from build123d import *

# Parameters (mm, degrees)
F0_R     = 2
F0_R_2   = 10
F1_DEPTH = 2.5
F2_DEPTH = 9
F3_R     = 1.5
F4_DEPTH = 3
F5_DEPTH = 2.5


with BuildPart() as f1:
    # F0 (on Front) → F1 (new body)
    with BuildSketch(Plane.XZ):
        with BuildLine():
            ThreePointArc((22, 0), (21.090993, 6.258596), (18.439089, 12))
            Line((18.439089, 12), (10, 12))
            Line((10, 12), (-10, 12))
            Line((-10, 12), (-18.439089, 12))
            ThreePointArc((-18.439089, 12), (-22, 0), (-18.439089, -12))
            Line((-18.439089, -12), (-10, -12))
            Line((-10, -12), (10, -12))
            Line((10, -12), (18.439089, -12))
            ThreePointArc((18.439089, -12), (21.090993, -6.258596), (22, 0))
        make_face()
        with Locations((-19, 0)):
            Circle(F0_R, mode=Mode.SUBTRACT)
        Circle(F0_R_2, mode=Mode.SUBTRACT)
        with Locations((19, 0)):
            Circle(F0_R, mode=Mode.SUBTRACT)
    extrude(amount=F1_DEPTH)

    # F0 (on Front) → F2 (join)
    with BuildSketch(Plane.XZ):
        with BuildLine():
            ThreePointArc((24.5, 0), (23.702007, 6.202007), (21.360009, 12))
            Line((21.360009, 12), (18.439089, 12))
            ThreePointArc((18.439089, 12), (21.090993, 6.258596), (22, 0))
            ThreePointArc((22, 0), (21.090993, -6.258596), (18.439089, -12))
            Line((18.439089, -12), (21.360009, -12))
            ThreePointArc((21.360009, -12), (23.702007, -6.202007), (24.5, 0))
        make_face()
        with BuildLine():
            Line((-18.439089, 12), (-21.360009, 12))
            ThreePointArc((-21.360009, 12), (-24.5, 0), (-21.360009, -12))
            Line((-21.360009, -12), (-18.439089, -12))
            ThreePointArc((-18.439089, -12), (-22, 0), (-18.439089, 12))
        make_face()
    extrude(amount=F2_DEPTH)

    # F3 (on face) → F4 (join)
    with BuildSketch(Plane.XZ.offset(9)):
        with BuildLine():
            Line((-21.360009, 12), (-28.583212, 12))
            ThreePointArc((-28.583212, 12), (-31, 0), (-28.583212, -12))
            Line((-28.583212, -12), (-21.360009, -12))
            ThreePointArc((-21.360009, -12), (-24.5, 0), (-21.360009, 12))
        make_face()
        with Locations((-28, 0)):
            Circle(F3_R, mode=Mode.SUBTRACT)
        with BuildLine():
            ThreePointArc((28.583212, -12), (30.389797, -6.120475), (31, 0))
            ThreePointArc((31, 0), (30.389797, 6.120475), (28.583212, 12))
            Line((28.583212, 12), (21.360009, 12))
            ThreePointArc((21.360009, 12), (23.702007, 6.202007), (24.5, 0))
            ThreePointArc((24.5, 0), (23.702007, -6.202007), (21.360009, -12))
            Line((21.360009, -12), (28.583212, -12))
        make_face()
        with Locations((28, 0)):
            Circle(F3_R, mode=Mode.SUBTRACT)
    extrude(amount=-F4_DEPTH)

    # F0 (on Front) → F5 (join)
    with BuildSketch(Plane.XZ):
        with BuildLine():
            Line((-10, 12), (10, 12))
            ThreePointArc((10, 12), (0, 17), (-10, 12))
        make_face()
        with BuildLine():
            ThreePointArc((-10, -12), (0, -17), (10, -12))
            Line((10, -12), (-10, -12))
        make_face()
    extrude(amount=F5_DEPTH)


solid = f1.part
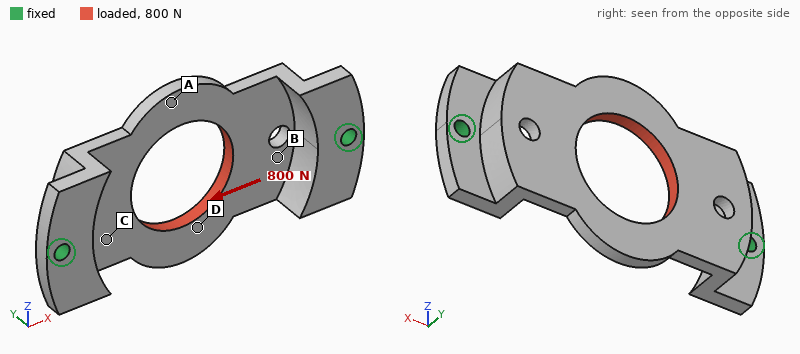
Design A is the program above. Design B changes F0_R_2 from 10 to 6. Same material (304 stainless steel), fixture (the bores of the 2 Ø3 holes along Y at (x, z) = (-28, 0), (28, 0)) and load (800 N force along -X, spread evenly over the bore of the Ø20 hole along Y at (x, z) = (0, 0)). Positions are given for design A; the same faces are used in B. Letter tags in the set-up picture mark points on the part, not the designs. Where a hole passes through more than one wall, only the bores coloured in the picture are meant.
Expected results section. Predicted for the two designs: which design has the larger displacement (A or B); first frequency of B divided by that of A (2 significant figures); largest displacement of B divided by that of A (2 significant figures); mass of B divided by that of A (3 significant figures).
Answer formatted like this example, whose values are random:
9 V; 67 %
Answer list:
A; 0.97; 0.88; 1.12
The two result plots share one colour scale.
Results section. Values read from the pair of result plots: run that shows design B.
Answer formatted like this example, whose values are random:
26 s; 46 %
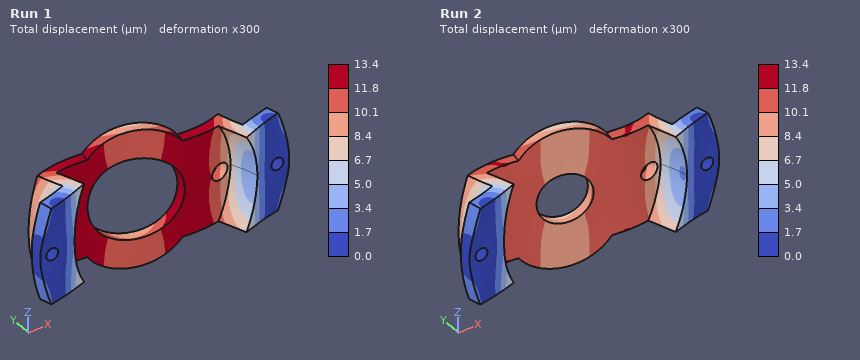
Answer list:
Run 2
